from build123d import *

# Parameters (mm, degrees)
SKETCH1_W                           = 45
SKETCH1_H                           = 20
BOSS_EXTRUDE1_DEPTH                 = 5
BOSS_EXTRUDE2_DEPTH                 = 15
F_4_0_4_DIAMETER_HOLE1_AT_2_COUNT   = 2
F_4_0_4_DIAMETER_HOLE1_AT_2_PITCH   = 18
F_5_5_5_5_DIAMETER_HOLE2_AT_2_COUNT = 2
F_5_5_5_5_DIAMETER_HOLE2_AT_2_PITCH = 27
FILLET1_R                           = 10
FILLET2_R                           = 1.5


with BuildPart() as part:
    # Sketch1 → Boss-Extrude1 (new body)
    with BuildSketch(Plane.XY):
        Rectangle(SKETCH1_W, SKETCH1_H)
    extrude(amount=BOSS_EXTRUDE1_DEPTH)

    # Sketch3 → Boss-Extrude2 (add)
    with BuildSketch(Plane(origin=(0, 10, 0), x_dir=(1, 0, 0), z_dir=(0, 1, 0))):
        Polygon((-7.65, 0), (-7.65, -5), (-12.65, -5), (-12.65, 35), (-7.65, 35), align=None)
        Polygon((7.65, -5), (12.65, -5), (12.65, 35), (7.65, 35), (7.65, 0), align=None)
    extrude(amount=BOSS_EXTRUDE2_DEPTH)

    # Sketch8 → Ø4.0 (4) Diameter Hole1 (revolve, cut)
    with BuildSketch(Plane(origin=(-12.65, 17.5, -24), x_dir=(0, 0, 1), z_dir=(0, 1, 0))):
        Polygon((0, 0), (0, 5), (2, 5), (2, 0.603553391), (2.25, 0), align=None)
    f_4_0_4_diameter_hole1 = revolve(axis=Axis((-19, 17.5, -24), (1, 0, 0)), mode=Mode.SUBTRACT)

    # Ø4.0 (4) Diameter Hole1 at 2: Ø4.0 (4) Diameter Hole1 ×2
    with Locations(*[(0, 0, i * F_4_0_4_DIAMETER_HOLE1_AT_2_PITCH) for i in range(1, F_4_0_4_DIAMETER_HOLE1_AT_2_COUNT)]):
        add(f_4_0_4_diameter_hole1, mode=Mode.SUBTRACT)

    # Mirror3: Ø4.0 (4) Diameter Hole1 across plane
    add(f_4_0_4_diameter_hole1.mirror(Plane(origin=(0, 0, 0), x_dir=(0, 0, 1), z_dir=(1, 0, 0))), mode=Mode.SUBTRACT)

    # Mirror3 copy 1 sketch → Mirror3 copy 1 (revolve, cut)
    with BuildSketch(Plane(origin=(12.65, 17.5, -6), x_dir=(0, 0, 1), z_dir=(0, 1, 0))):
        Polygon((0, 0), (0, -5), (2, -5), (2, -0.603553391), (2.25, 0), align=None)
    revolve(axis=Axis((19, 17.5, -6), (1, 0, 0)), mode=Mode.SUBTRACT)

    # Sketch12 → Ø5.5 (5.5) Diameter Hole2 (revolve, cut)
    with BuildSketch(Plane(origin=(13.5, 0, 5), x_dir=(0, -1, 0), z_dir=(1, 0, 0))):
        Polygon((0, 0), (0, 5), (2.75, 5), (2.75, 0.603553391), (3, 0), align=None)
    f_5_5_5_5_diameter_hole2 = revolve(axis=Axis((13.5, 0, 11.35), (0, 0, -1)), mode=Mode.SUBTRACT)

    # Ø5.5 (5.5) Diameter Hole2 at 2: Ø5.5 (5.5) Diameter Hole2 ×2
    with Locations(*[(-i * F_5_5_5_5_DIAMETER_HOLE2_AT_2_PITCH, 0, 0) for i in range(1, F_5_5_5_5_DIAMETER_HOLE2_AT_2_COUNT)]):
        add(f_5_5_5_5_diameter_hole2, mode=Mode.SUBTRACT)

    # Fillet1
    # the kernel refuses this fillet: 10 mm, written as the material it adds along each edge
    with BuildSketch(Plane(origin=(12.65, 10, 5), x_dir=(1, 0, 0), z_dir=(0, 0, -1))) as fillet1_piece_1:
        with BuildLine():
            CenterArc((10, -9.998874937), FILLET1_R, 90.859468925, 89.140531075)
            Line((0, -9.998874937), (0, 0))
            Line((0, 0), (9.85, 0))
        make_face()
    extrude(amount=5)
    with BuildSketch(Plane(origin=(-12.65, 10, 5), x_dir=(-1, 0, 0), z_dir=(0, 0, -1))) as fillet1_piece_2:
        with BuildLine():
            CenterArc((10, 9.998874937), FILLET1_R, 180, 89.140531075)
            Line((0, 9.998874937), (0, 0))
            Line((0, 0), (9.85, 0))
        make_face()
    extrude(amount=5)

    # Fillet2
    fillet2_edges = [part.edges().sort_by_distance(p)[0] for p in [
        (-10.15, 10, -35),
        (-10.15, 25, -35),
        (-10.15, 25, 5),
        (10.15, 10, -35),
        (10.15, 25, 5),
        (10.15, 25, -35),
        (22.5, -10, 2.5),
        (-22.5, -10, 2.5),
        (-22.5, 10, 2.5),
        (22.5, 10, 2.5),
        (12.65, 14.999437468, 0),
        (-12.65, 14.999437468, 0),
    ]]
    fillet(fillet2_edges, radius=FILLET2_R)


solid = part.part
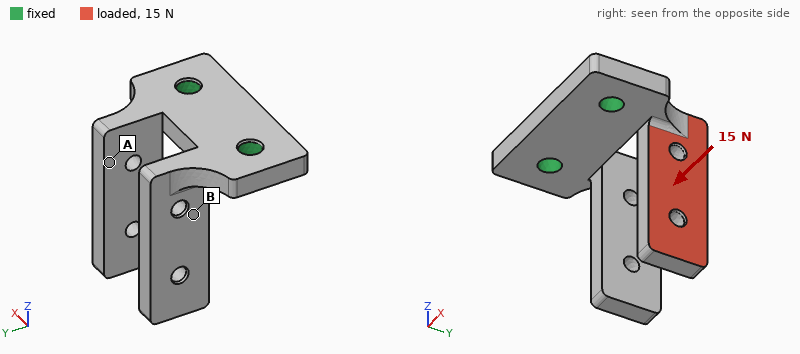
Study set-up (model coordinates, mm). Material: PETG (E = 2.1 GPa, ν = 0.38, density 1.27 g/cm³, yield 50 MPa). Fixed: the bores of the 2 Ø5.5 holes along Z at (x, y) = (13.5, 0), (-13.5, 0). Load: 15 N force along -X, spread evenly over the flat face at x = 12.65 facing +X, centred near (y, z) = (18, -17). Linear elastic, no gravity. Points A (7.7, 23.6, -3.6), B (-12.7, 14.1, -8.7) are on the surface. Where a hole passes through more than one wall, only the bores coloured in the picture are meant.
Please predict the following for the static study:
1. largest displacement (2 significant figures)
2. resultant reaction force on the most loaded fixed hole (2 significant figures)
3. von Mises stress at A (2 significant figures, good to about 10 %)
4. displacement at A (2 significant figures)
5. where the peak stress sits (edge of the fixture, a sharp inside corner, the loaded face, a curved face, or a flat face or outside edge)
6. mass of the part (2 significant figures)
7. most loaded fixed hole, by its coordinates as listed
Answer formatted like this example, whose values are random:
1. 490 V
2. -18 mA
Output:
1. 0.71 mm
2. 13 N
3. 2.8 MPa
4. 0.11 mm
5. a sharp inside corner
6. 13 g
7. (13.5, 0)
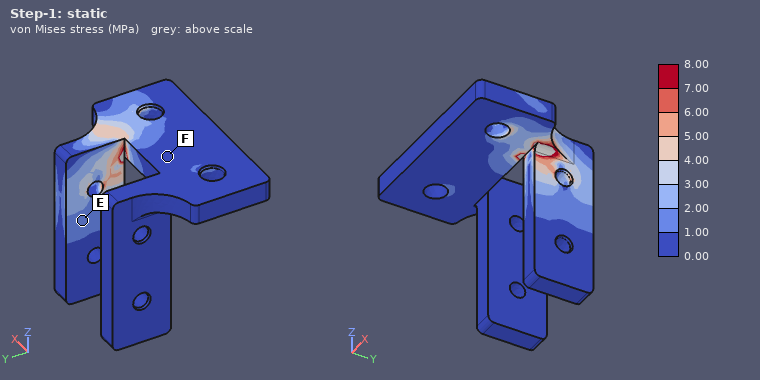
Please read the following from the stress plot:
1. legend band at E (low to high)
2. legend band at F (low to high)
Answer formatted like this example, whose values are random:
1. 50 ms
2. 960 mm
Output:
1. 1.00 to 2.00 MPa
2. 0.00 to 1.00 MPa
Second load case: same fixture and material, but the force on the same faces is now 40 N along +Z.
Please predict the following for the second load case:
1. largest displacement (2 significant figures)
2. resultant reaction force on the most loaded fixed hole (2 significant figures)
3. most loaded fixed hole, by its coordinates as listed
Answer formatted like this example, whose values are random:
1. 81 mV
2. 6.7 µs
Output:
1. 0.75 mm
2. 41 N
3. (13.5, 0)
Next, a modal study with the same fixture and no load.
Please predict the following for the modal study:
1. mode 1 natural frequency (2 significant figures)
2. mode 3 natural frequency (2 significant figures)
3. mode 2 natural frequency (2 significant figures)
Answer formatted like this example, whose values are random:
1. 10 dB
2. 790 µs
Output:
1. 490 Hz
2. 530 Hz
3. 510 Hz
